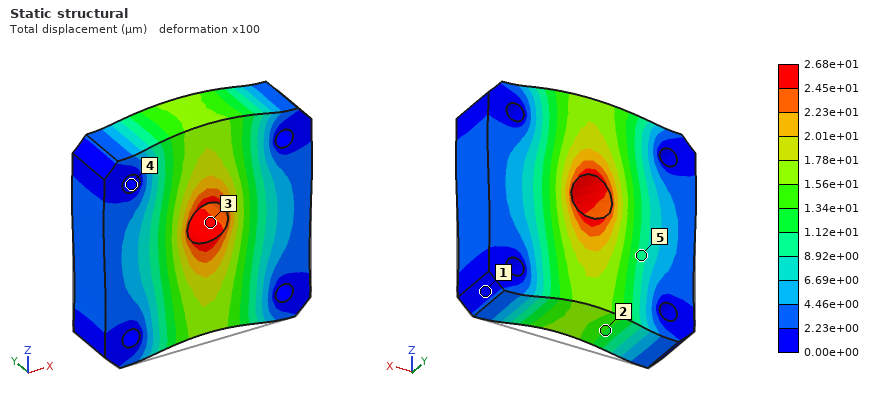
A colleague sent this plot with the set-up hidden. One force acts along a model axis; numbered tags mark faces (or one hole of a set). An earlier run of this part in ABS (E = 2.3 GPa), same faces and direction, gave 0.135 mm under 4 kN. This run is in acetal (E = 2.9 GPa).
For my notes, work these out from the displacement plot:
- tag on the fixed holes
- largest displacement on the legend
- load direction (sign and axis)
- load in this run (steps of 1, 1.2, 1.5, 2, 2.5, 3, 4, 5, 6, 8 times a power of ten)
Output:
4
2.68e+01 µm
+Z
1 kN
